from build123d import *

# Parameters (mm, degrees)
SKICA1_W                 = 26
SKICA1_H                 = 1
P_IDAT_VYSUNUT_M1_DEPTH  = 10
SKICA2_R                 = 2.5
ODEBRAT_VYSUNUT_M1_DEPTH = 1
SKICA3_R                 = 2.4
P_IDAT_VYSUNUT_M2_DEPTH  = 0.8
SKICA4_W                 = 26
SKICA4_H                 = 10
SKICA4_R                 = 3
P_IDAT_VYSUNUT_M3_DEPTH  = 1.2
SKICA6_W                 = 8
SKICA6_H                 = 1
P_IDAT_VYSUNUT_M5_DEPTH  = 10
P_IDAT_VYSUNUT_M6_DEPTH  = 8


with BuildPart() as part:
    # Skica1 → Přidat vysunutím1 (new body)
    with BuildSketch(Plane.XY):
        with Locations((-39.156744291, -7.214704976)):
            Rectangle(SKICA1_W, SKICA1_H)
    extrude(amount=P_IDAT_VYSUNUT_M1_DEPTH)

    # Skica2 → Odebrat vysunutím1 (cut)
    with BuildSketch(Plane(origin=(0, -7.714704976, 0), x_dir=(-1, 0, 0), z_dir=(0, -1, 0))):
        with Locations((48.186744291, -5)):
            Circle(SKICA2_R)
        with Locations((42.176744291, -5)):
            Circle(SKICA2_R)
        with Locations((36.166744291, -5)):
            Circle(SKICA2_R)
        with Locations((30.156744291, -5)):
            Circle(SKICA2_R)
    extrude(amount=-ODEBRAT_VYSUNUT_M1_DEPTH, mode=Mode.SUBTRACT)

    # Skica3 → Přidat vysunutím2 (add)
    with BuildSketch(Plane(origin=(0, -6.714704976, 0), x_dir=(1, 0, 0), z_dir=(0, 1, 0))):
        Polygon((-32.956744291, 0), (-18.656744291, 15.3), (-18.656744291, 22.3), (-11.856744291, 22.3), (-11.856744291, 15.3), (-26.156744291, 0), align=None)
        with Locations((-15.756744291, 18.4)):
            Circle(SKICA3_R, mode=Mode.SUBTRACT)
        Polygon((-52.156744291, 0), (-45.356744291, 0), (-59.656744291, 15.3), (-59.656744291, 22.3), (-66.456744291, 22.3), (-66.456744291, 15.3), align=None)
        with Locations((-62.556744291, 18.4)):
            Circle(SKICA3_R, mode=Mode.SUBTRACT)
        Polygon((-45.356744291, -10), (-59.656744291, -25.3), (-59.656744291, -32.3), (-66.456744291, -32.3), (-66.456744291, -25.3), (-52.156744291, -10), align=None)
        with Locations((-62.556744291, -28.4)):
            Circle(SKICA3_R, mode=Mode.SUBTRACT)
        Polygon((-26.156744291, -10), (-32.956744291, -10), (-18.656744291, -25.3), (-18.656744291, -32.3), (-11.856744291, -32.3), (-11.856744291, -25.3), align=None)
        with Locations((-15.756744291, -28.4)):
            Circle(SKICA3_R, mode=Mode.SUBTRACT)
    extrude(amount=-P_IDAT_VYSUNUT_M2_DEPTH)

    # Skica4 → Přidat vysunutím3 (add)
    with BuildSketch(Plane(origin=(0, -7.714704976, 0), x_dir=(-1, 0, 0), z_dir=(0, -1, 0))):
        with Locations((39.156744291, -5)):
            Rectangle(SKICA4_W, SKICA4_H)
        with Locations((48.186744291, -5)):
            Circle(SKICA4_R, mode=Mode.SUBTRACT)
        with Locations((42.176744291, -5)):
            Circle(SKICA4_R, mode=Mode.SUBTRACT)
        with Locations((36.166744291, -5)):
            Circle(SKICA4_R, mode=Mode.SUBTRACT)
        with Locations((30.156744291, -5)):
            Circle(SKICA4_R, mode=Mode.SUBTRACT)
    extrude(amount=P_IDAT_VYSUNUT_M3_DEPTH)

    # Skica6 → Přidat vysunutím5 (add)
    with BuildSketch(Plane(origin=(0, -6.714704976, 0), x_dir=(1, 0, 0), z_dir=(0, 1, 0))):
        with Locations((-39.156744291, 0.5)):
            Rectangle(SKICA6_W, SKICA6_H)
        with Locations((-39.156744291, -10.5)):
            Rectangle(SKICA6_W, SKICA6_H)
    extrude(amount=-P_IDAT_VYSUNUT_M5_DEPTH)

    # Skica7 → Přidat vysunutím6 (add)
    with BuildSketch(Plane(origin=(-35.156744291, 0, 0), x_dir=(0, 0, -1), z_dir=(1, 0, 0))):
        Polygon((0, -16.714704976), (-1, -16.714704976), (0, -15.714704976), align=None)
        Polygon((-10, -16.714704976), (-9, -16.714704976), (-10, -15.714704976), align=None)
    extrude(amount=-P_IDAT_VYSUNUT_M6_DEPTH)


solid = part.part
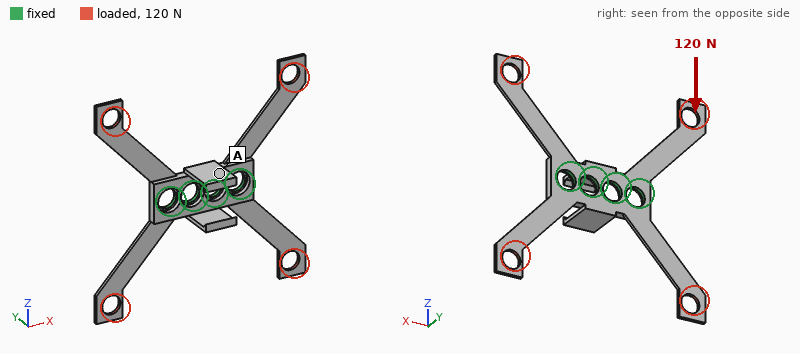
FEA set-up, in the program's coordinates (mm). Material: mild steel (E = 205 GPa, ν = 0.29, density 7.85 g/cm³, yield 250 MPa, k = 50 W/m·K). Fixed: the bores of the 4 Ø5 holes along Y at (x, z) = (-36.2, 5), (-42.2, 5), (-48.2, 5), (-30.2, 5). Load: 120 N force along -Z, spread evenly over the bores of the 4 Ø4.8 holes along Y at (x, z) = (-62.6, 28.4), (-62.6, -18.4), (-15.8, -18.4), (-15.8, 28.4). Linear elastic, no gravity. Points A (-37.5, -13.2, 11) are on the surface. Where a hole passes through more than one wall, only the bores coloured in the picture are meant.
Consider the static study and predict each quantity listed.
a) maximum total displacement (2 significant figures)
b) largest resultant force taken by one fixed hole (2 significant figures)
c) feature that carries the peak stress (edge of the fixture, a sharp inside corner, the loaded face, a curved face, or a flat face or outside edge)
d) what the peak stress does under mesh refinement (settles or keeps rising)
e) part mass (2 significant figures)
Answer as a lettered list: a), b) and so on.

a) 58 µm
b) 120 N
c) a sharp inside corner
d) keeps rising
e) 7.5 g
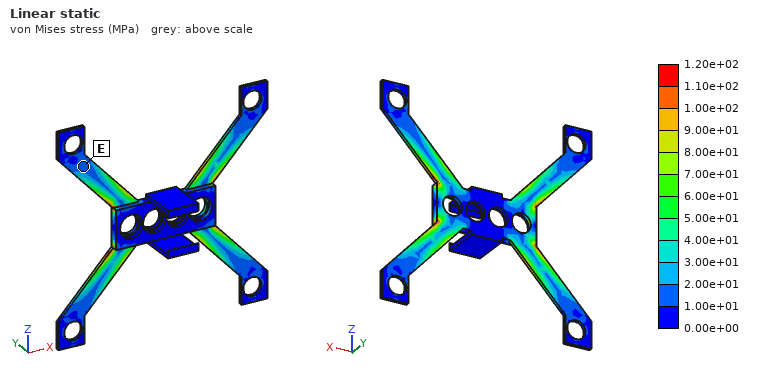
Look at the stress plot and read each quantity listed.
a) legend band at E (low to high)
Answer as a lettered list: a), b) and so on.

a) 1.00e+01 to 2.00e+01 MPa
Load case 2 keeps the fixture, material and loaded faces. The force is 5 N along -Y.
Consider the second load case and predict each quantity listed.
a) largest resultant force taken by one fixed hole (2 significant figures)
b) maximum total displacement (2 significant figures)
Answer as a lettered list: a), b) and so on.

a) 9.4 N
b) 0.15 mm
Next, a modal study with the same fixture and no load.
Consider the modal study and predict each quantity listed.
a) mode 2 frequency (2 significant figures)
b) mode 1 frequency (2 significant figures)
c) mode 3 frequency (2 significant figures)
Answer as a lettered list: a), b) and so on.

a) 940 Hz
b) 940 Hz
c) 940 Hz
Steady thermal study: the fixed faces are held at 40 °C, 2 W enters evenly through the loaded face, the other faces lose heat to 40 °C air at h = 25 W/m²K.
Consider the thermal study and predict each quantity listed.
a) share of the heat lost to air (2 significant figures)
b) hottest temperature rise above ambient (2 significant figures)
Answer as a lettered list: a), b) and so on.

a) 39 %
b) 49 K
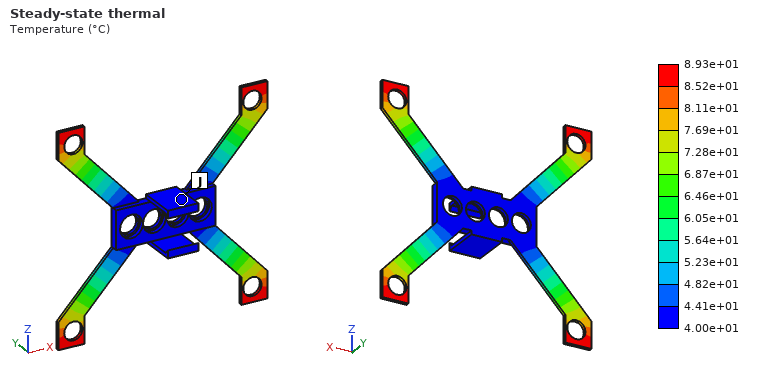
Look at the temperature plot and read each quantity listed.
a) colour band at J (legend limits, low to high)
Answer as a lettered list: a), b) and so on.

a) 4.00e+01 to 4.41e+01 °C
